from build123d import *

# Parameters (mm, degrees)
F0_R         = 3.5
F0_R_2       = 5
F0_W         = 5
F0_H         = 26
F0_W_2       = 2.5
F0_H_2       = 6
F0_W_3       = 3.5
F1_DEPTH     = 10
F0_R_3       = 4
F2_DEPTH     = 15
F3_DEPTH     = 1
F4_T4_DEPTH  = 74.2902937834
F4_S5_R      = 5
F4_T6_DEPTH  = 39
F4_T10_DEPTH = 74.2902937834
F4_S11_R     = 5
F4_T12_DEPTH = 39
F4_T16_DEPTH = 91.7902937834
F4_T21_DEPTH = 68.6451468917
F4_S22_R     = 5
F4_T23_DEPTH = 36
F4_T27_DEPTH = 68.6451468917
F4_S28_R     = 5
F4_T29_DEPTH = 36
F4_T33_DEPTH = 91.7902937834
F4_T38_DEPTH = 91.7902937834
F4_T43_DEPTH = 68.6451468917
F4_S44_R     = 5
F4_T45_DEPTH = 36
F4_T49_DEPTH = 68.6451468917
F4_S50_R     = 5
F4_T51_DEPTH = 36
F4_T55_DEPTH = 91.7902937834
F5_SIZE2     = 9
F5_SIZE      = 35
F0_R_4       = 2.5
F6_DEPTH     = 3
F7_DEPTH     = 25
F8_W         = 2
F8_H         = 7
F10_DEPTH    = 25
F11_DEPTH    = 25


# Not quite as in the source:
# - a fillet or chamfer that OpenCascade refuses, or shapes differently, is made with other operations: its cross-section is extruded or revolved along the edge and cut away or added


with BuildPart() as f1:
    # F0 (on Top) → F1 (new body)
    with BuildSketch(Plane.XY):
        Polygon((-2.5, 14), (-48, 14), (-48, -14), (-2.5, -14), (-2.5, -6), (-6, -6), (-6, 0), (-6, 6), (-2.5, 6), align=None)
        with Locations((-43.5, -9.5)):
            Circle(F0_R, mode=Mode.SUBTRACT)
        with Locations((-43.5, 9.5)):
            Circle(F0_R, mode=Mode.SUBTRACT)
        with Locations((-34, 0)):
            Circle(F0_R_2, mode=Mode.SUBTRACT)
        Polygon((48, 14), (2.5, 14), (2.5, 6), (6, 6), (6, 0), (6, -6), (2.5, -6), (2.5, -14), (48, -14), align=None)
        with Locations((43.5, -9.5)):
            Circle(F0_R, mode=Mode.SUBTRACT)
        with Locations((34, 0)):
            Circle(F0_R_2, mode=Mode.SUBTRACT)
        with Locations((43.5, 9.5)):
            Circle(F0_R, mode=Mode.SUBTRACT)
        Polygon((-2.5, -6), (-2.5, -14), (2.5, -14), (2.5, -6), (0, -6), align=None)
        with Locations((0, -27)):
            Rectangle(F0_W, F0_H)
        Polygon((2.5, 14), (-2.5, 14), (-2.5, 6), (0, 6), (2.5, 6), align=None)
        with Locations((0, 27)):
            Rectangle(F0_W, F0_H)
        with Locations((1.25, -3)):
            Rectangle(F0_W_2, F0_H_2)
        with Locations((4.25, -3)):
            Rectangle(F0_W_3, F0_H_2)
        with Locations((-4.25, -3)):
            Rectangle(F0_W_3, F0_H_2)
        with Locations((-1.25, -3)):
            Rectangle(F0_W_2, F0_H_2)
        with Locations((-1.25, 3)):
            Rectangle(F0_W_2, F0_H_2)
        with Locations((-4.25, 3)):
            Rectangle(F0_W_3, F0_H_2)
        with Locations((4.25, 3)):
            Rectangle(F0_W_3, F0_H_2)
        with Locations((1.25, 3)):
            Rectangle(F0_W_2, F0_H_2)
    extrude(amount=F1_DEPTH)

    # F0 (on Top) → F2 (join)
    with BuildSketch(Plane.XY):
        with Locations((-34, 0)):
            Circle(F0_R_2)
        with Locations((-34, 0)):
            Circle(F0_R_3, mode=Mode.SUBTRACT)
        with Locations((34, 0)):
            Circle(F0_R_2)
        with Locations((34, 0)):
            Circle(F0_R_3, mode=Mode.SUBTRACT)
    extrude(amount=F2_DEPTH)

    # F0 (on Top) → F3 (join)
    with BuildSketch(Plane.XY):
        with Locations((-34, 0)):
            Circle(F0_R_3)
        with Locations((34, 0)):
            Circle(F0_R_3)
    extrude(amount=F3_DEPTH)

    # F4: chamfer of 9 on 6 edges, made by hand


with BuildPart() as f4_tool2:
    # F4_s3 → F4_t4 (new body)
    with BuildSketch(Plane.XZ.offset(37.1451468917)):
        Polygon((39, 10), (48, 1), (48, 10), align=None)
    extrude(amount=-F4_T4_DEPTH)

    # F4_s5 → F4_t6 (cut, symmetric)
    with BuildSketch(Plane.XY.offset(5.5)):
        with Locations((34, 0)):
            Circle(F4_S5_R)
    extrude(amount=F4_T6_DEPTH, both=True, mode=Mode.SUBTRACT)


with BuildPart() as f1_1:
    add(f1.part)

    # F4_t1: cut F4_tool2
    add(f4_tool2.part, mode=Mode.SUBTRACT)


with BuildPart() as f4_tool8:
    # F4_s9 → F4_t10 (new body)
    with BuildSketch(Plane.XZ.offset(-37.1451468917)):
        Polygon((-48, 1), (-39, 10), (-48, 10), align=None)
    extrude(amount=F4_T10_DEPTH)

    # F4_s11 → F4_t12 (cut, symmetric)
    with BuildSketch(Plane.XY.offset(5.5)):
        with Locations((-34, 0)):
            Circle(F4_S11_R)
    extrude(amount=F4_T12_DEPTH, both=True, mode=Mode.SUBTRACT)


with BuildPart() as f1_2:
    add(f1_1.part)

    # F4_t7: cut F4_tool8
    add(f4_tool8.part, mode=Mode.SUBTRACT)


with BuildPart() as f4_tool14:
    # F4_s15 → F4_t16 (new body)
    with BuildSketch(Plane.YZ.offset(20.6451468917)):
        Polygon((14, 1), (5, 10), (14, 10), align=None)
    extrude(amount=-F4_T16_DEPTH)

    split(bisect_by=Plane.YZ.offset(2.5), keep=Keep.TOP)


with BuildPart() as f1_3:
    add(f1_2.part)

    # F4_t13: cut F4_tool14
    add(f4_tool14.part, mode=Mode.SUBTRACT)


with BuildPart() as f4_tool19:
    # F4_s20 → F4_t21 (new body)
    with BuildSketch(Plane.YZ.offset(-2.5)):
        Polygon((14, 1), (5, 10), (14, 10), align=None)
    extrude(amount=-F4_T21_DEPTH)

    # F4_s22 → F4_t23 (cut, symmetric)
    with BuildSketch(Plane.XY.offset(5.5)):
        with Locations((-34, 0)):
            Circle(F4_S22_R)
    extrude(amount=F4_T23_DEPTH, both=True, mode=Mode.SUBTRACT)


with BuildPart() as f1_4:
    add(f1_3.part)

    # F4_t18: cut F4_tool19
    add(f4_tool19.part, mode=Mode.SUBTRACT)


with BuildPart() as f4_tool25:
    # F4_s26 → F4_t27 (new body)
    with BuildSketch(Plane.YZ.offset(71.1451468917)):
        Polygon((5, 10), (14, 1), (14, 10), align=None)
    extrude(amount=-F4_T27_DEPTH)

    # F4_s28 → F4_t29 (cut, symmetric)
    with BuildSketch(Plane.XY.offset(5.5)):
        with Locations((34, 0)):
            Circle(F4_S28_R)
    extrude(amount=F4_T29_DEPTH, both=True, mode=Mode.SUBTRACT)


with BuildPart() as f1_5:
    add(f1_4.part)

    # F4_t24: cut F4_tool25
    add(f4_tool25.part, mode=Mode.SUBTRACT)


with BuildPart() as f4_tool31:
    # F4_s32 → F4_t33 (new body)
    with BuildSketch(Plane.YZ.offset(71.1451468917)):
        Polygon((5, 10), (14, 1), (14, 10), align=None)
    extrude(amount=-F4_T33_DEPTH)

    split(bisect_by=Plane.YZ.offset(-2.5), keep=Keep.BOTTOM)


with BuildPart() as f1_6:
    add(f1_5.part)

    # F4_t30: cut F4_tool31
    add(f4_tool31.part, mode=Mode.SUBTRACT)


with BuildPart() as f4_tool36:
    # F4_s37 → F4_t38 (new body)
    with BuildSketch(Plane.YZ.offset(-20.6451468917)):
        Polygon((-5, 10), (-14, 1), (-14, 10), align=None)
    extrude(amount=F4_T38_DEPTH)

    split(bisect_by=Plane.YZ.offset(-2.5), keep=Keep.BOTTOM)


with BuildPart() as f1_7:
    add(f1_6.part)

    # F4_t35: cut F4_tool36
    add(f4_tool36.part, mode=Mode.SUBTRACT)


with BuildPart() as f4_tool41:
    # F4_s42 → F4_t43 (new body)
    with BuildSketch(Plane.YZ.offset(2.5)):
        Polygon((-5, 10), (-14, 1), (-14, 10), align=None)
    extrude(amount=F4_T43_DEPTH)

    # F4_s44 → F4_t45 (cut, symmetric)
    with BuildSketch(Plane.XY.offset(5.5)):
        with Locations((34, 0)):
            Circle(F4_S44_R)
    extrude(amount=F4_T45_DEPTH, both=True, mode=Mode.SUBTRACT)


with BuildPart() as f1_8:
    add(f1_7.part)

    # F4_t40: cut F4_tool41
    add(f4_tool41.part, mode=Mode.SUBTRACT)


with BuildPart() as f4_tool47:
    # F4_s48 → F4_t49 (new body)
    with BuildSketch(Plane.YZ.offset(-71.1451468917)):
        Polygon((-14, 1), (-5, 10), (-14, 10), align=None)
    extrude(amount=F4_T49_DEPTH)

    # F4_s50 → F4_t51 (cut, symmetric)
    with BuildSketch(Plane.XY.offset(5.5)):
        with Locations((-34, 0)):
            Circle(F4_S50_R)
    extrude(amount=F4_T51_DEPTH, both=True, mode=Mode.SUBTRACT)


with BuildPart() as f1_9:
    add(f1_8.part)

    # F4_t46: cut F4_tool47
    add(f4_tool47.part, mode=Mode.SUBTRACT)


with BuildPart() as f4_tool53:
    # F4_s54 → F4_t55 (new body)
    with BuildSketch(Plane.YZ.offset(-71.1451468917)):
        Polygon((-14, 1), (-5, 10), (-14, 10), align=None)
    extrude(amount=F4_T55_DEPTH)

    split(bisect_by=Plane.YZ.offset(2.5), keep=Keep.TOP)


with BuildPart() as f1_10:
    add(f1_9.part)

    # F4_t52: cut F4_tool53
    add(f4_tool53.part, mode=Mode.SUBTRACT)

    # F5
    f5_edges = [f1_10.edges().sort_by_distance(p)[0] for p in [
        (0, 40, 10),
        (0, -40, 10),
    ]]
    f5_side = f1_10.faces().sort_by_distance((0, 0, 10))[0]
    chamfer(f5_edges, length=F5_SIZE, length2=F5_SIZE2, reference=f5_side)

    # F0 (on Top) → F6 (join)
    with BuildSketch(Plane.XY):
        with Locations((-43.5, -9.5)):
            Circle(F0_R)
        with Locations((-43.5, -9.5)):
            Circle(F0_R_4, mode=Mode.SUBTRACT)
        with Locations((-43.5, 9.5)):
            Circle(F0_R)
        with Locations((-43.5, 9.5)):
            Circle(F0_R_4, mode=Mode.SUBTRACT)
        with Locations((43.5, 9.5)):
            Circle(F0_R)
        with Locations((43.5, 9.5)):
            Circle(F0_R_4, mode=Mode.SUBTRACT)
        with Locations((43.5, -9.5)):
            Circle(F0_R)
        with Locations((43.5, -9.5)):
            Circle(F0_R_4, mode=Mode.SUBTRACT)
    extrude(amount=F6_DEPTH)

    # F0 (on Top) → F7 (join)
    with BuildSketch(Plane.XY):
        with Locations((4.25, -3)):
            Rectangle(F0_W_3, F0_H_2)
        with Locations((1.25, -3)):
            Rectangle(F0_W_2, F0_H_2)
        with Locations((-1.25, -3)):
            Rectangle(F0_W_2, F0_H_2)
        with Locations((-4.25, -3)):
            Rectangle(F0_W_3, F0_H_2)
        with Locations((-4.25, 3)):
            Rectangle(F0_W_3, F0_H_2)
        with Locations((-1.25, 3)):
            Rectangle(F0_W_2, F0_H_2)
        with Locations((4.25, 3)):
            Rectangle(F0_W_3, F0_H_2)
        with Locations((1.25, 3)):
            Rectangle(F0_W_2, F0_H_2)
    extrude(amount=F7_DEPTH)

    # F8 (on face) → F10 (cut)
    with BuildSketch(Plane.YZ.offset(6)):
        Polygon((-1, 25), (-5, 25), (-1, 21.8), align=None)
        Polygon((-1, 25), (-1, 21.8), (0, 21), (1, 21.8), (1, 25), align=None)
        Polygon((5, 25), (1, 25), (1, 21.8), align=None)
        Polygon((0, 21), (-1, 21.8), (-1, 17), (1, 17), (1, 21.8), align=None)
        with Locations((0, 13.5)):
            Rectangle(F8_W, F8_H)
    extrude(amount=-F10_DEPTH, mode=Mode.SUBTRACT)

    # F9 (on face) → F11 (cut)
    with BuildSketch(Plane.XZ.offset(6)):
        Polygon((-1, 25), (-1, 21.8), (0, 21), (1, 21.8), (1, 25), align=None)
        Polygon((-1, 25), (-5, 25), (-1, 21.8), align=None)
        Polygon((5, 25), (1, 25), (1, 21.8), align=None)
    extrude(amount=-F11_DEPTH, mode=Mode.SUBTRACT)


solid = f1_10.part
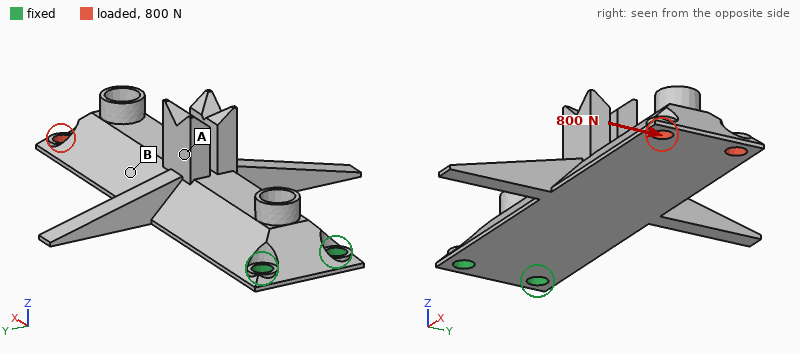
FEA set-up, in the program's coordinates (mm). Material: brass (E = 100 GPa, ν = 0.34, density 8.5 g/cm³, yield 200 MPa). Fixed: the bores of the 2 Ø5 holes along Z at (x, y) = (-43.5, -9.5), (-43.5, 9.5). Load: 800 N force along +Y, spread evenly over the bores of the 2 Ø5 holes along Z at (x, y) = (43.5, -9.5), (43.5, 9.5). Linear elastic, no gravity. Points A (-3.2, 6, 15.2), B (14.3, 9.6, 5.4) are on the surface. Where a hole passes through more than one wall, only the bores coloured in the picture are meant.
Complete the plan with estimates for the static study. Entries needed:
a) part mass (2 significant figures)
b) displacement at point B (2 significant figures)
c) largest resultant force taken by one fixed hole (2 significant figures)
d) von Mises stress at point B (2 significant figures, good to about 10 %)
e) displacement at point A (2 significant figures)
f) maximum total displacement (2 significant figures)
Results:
170 g
0.13 mm
3.5 kN
28 MPa
0.059 mm
0.28 mm
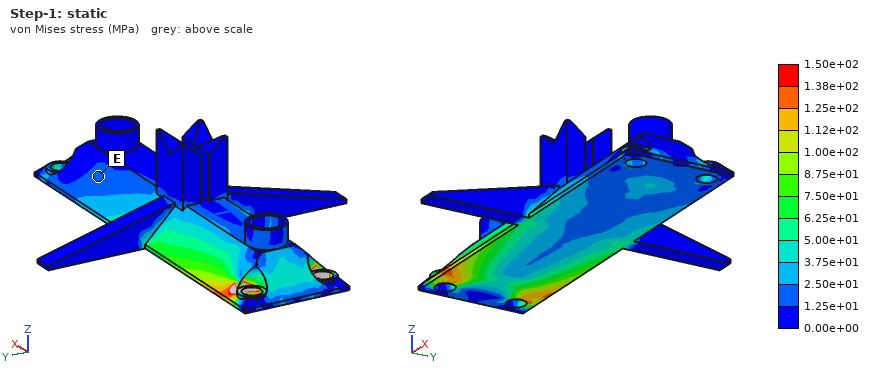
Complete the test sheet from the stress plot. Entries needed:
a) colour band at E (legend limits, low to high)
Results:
1.25e+01 to 2.50e+01 MPa
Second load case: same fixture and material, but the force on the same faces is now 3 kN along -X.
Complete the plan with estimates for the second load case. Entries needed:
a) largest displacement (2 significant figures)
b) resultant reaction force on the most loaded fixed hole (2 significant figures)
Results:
0.21 mm
1.5 kN
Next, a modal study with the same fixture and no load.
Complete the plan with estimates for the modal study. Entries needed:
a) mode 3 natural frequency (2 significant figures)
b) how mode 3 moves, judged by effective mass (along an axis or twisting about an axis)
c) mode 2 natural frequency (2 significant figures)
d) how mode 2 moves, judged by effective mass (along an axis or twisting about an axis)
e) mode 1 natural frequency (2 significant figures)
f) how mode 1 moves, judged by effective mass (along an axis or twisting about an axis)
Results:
2400 Hz
twisting about X
1400 Hz
along Y
380 Hz
along Z
